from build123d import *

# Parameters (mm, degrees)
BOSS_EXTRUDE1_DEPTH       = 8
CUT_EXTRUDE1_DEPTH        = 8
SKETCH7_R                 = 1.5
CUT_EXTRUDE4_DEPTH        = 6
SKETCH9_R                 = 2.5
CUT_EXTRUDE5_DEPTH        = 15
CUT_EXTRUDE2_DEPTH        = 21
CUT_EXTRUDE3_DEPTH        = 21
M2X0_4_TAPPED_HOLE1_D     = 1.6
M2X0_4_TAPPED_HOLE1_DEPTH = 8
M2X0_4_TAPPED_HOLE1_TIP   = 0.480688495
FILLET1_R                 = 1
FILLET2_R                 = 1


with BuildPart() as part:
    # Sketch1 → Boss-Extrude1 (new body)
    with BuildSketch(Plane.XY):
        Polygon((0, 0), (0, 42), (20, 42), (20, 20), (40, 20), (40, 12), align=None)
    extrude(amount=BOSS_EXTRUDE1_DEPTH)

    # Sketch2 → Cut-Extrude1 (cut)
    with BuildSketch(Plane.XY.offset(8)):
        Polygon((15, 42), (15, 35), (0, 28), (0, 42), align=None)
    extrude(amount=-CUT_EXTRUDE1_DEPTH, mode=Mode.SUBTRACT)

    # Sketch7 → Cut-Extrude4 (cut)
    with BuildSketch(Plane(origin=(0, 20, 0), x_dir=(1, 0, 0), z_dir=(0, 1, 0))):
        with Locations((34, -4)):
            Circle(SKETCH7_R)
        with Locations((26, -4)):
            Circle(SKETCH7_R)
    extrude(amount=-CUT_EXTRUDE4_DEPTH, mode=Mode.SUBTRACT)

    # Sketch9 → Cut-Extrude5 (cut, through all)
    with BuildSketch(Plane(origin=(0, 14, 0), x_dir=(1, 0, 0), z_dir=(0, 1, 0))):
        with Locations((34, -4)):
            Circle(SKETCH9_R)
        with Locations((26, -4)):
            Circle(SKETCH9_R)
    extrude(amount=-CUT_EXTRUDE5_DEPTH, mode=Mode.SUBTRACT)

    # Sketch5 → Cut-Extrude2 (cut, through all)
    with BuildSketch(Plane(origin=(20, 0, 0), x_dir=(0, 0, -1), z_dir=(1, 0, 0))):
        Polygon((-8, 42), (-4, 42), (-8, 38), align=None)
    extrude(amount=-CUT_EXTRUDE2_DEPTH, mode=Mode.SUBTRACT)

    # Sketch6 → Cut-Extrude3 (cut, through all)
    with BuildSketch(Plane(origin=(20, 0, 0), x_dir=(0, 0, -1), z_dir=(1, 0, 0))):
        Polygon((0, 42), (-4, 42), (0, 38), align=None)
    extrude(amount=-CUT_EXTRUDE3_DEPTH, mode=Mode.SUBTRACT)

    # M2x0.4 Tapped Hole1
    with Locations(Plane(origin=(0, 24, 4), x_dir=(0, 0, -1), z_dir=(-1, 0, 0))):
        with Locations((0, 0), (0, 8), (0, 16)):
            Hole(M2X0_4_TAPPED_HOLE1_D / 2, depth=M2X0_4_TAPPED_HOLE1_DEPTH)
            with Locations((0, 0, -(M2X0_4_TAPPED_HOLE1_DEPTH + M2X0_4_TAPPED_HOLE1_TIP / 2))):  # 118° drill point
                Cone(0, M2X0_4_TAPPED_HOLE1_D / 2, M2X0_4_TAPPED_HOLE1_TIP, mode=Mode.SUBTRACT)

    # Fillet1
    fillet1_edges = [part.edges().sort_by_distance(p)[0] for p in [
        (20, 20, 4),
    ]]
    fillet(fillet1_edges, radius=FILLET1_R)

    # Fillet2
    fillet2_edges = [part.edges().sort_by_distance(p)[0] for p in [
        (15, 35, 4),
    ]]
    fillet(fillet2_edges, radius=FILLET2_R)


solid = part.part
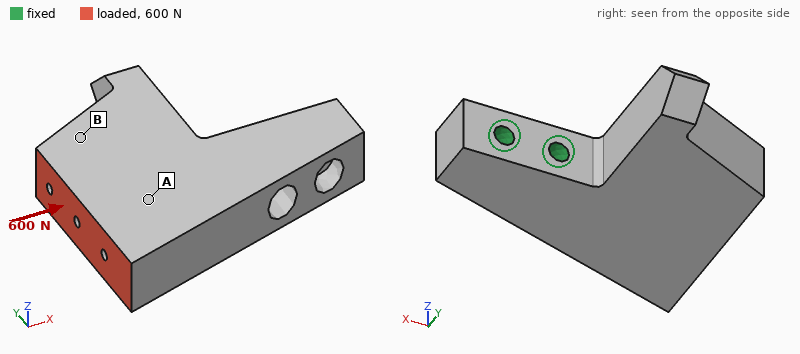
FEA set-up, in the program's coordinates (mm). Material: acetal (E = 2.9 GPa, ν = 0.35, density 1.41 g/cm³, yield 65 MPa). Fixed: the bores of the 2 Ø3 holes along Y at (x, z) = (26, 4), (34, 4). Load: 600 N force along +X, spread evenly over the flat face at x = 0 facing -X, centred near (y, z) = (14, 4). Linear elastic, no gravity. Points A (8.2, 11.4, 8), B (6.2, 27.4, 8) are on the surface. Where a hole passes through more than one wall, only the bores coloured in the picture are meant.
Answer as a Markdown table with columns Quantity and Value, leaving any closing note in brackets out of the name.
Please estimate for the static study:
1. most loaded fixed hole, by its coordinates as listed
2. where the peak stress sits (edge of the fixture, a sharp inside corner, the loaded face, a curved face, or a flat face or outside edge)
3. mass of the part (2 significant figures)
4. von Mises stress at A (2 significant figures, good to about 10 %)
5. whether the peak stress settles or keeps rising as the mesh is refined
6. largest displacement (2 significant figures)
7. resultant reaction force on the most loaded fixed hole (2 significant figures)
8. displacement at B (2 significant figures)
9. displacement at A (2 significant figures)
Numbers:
| Quantity | Value |
|---|---|
| most loaded fixed hole, by its coordinates as listed | (26, 4) |
| where the peak stress sits | edge of the fixture |
| mass of the part | 8.9 g |
| von Mises stress at A | 3.4 MPa |
| whether the peak stress settles or keeps rising as the mesh is refined | keeps rising |
| largest displacement | 0.19 mm |
| resultant reaction force on the most loaded fixed hole | 470 N |
| displacement at B | 0.080 mm |
| displacement at A | 0.097 mm |
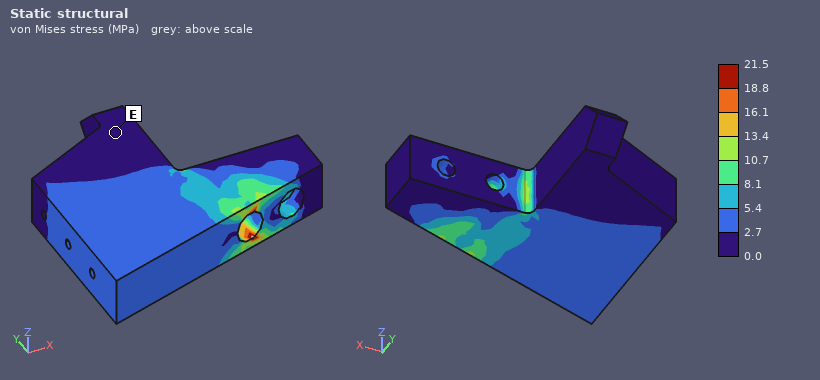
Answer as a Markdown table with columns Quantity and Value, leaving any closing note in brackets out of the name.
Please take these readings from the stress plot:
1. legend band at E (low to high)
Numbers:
| Quantity | Value |
|---|---|
| legend band at E | 0.0 to 2.7 MPa |
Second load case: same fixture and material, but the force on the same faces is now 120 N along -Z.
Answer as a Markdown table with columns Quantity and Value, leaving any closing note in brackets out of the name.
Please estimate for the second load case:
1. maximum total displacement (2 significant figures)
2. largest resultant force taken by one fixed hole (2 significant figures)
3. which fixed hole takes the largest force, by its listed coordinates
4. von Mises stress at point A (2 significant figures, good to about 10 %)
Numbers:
| Quantity | Value |
|---|---|
| maximum total displacement | 0.66 mm |
| largest resultant force taken by one fixed hole | 300 N |
| which fixed hole takes the largest force, by its listed coordinates | (26, 4) |
| von Mises stress at point A | 4.0 MPa |
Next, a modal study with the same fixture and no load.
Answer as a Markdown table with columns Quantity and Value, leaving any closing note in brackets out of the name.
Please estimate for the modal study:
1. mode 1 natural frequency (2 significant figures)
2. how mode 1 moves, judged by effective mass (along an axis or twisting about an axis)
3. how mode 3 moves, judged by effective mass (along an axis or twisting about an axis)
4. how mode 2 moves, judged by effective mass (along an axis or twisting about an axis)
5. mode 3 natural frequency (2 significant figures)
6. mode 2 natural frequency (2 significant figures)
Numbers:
| Quantity | Value |
|---|---|
| mode 1 natural frequency | 1400 Hz |
| how mode 1 moves, judged by effective mass | along Z |
| how mode 3 moves, judged by effective mass | twisting about X |
| how mode 2 moves, judged by effective mass | along Y |
| mode 3 natural frequency | 1900 Hz |
| mode 2 natural frequency | 1600 Hz |
